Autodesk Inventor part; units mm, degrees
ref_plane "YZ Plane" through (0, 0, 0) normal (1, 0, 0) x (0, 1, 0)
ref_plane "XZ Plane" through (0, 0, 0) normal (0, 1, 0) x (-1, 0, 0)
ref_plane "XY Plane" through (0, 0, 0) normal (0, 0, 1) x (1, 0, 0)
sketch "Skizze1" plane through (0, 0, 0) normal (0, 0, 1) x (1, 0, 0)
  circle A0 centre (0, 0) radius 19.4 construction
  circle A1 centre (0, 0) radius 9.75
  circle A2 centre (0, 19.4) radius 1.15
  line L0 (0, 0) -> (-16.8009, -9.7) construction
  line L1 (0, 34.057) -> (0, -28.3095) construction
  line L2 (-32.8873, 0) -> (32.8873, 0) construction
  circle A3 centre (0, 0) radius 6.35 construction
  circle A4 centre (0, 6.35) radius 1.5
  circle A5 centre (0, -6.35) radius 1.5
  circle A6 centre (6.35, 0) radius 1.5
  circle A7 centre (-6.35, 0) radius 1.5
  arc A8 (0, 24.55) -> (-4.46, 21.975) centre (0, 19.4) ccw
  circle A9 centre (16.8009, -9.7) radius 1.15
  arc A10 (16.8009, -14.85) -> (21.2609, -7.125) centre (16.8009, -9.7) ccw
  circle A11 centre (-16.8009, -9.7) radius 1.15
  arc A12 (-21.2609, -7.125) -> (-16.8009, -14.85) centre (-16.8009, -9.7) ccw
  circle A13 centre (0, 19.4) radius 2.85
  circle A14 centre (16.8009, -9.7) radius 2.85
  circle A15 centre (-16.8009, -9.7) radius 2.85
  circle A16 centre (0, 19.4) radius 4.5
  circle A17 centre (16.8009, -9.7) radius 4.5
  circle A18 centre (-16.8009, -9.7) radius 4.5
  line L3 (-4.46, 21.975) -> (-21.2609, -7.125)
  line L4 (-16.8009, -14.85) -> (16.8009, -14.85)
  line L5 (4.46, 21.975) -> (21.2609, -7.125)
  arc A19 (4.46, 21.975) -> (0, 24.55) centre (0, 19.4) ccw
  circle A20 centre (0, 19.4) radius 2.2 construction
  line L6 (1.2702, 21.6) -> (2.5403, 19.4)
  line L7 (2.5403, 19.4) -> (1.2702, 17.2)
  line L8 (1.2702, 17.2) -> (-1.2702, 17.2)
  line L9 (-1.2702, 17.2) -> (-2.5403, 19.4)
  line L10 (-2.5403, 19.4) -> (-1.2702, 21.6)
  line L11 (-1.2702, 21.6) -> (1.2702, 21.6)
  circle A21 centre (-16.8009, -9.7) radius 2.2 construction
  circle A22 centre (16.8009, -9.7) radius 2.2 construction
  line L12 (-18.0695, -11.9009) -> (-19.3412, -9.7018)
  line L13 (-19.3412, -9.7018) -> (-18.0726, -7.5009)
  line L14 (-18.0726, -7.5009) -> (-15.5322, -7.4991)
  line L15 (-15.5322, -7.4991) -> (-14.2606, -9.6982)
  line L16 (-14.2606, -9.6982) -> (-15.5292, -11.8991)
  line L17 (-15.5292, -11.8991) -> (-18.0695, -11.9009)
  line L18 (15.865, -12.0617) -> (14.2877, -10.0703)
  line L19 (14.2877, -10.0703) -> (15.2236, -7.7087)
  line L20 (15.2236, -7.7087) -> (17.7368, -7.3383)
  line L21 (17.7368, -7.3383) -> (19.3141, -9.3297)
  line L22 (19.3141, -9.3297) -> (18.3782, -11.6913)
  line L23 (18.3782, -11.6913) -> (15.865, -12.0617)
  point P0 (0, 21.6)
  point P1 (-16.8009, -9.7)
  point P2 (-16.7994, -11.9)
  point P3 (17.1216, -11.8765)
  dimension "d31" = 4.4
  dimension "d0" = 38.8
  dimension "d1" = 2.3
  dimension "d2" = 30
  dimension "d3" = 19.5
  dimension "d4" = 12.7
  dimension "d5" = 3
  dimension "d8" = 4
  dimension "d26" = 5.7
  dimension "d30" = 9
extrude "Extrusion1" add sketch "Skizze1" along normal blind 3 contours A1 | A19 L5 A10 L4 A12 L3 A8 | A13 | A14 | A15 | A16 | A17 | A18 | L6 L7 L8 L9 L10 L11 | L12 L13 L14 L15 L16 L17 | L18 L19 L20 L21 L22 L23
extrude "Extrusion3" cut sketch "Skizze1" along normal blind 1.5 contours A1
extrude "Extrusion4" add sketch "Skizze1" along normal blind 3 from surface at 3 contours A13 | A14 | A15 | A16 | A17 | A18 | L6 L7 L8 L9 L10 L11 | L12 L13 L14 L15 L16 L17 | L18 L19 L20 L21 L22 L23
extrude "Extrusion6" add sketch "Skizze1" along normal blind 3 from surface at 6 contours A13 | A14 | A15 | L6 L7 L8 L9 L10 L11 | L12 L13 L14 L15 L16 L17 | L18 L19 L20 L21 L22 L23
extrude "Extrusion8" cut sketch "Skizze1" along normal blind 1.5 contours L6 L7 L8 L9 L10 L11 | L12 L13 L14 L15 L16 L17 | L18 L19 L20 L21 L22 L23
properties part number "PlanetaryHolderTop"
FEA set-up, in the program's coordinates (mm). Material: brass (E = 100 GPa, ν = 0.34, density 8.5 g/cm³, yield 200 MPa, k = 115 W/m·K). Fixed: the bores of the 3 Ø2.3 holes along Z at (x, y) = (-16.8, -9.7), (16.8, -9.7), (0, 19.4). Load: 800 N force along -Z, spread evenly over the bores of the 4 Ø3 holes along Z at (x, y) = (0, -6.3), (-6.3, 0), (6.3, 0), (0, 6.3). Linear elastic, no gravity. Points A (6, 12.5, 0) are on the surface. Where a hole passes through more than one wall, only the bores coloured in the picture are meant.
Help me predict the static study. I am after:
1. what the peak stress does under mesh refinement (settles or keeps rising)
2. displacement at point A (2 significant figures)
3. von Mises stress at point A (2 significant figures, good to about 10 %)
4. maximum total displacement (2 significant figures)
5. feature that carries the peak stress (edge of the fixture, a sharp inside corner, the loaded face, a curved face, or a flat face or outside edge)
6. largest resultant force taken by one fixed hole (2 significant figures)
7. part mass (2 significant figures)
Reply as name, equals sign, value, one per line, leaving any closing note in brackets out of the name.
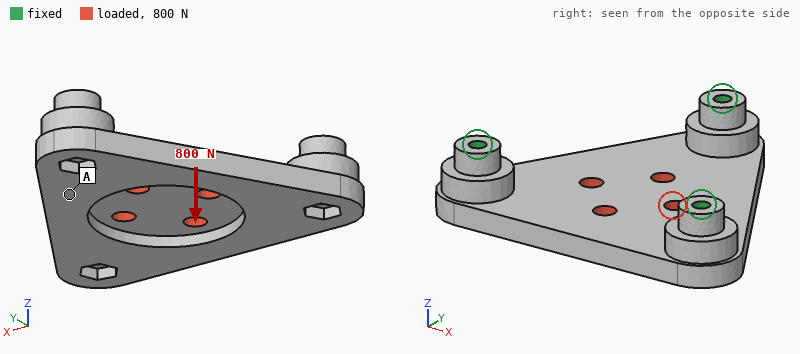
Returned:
what the peak stress does under mesh refinement = keeps rising
displacement at point A = 10.0 µm
von Mises stress at point A = 41 MPa
maximum total displacement = 50 µm
feature that carries the peak stress = a sharp inside corner
largest resultant force taken by one fixed hole = 290 N
part mass = 29 g
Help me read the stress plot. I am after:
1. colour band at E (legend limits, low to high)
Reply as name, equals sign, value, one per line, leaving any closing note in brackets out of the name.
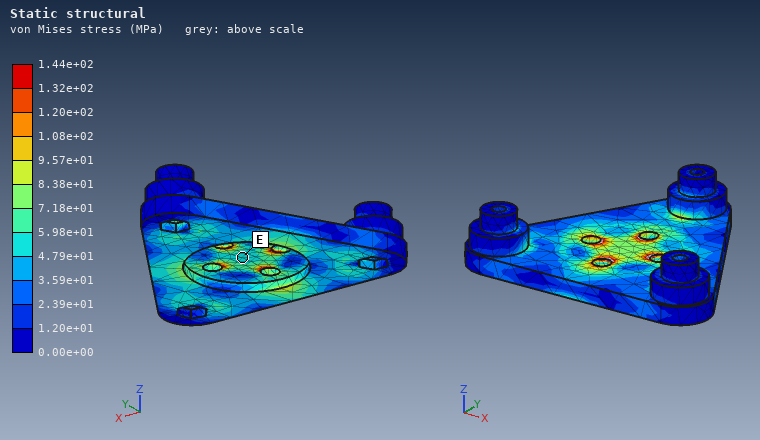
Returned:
colour band at E = 4.79e+01 to 5.98e+01 MPa
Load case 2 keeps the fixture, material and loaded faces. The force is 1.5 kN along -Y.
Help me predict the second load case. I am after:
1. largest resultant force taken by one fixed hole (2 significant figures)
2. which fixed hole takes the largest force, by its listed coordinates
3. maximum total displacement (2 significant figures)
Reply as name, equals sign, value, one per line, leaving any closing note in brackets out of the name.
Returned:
largest resultant force taken by one fixed hole = 650 N
which fixed hole takes the largest force, by its listed coordinates = (0, 19.4)
maximum total displacement = 7.2 µm
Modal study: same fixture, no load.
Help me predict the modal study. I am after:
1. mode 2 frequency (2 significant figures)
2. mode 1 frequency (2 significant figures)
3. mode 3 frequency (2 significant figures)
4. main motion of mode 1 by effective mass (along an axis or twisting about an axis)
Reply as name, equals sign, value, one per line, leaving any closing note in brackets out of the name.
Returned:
mode 2 frequency = 12 kHz
mode 1 frequency = 10 kHz
mode 3 frequency = 12 kHz
main motion of mode 1 by effective mass = along Z
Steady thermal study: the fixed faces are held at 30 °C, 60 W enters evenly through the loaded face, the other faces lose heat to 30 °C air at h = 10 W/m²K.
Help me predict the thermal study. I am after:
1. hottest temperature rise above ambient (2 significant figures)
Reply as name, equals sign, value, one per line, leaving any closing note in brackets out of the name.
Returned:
hottest temperature rise above ambient = 81 K
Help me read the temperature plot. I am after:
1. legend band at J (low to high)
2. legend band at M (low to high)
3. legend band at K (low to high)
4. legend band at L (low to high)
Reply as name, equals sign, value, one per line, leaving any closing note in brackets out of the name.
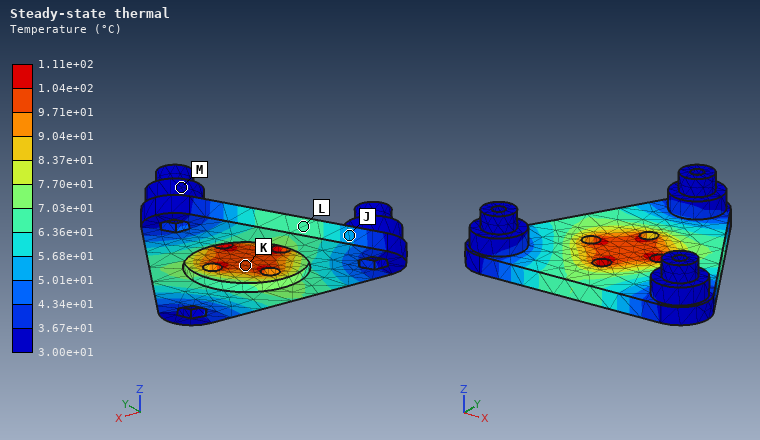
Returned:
legend band at J = 5.01e+01 to 5.68e+01 °C
legend band at M = 3.00e+01 to 3.67e+01 °C
legend band at K = 9.71e+01 to 1.04e+02 °C
legend band at L = 6.36e+01 to 7.03e+01 °C
